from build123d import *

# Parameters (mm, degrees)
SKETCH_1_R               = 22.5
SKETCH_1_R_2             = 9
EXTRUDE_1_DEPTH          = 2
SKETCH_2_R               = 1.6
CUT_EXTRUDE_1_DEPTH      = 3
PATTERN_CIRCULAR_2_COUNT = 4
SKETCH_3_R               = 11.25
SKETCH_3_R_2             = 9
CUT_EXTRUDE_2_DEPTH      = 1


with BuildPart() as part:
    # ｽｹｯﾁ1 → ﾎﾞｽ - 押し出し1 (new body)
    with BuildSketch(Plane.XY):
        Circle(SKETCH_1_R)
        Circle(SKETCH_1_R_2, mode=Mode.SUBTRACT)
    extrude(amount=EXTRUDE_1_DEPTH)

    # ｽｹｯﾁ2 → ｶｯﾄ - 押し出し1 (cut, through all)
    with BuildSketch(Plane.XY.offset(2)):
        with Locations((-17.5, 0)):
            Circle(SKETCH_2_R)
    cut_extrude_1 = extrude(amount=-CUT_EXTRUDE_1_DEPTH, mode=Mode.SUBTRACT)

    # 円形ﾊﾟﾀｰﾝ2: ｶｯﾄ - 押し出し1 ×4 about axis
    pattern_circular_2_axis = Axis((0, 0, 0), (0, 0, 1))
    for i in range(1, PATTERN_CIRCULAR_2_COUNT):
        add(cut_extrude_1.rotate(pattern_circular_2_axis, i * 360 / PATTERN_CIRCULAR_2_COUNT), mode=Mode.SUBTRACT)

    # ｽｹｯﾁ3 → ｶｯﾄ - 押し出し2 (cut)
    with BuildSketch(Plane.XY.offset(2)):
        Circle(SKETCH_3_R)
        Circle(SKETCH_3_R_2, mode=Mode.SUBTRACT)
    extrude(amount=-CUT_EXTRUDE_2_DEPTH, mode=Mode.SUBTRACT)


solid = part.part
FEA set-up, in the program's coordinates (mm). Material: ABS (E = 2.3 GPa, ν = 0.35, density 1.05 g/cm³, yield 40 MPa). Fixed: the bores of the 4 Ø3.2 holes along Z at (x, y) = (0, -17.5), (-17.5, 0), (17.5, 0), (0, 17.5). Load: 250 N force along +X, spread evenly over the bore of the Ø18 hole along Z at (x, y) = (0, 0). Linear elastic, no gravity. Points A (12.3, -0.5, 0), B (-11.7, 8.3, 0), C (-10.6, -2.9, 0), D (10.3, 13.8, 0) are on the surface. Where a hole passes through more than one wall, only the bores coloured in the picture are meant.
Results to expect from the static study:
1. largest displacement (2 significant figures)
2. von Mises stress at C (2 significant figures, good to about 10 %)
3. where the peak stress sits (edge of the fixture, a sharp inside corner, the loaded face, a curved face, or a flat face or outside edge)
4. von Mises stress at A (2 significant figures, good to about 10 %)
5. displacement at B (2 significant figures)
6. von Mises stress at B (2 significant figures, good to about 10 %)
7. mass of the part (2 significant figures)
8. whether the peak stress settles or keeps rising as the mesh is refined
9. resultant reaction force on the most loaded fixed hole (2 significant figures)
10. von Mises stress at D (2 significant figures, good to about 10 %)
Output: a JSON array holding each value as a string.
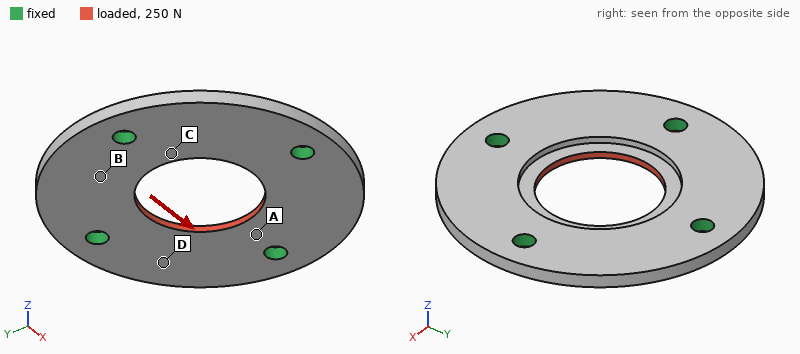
["37 µm", "5.9 MPa", "edge of the fixture", "6.7 MPa", "18 µm", "2.6 MPa", "2.6 g", "keeps rising", "67 N", "1.4 MPa"]
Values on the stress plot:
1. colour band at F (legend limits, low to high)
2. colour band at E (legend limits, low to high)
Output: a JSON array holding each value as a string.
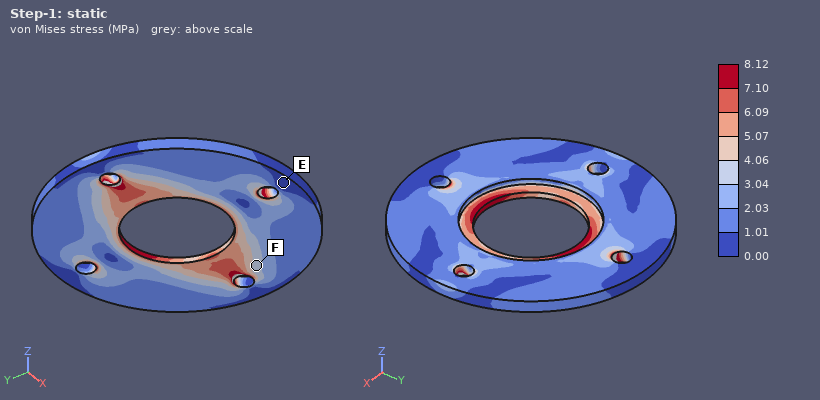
["3.04 to 4.06 MPa", "0.00 to 1.01 MPa"]
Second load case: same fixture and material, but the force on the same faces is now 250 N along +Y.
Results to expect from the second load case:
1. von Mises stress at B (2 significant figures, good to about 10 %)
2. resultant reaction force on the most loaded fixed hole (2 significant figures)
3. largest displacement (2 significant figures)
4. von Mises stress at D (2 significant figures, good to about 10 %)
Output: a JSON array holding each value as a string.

["2.0 MPa", "67 N", "37 µm", "1.4 MPa"]
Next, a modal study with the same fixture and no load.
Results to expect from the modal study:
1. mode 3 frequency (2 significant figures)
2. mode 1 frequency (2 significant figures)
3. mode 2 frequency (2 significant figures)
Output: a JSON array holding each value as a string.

["3800 Hz", "3700 Hz", "3800 Hz"]
